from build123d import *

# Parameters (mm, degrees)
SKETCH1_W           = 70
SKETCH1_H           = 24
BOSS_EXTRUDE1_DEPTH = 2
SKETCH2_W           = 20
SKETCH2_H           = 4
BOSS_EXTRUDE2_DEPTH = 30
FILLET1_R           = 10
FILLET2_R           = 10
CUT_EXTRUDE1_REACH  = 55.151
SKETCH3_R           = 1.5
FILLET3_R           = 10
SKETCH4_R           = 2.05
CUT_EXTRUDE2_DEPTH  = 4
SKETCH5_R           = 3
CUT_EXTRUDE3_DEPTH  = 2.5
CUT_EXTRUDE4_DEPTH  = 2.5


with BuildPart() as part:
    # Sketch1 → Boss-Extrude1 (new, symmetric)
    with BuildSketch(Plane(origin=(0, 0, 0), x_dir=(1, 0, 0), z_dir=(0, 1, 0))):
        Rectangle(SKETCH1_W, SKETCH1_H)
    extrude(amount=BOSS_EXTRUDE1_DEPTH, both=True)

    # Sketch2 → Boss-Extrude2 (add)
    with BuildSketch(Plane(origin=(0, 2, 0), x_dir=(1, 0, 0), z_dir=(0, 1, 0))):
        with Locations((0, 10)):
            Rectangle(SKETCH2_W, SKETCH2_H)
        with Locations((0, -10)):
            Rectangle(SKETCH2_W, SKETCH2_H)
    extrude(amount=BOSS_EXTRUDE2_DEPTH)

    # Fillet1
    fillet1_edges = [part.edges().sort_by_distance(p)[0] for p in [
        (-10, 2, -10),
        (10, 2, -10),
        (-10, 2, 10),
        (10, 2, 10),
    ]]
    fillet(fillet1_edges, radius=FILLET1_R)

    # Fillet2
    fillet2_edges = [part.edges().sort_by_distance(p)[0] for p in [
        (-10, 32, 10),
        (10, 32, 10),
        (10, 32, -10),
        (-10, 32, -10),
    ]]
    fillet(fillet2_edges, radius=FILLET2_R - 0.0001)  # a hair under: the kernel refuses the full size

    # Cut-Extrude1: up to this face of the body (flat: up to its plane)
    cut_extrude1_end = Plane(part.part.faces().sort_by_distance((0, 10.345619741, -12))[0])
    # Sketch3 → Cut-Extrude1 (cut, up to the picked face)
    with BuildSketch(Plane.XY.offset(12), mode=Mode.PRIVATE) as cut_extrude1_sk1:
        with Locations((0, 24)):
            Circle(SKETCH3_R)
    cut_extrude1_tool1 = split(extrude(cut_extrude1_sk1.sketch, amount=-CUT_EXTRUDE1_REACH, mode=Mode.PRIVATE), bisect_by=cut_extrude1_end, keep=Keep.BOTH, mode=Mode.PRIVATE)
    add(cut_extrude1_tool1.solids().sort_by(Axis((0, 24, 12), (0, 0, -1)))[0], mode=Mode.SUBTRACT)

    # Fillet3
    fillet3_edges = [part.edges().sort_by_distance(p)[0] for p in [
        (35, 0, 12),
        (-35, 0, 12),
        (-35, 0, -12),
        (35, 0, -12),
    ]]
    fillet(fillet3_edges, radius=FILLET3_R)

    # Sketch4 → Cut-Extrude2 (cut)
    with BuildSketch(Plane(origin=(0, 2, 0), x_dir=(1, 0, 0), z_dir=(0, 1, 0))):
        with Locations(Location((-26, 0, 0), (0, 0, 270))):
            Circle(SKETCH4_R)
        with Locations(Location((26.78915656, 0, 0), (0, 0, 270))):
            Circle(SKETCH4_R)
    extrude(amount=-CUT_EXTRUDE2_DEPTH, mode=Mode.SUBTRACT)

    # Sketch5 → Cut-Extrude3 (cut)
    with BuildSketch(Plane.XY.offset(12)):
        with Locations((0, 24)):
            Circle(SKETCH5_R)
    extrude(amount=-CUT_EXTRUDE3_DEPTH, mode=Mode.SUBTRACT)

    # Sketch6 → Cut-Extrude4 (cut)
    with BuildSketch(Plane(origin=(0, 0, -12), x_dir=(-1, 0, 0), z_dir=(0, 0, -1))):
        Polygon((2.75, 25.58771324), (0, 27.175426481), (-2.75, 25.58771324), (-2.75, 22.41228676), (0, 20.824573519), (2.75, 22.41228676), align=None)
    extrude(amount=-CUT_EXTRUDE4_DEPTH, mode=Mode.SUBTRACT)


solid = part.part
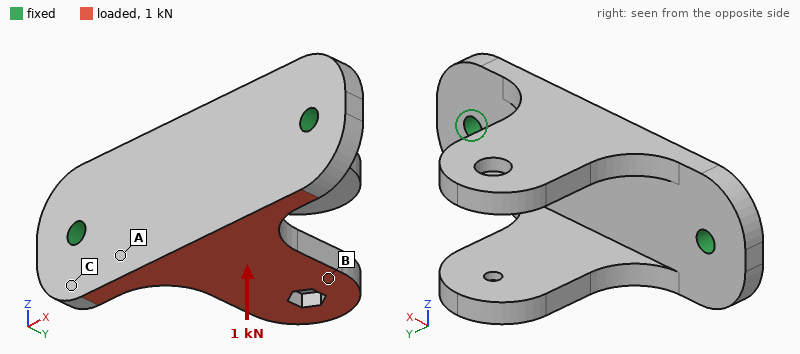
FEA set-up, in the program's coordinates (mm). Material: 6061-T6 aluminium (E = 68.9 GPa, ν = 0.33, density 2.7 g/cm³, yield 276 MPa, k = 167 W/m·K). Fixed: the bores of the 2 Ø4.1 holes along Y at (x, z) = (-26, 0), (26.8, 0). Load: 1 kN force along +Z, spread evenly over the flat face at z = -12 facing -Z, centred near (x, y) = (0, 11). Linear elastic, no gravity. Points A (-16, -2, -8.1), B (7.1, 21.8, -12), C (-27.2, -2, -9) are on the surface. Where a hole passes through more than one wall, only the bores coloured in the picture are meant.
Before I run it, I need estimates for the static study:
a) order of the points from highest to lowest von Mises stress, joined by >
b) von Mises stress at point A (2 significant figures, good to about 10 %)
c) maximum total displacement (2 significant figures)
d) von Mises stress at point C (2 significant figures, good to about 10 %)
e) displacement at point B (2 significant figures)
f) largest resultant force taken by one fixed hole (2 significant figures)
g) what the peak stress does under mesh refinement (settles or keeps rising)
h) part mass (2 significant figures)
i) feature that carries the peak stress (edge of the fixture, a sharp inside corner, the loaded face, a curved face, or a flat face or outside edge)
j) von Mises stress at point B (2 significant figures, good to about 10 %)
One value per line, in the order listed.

A > C > B
78 MPa
0.59 mm
50 MPa
0.38 mm
510 N
keeps rising
29 g
edge of the fixture
20 MPa
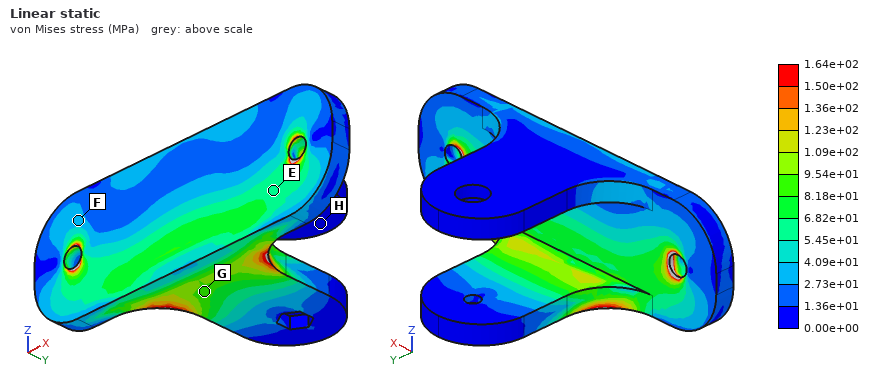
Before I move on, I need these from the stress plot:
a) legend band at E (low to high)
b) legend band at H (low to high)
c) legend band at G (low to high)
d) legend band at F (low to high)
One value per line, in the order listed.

5.45e+01 to 6.82e+01 MPa
0.00e+00 to 1.36e+01 MPa
8.18e+01 to 9.54e+01 MPa
2.73e+01 to 4.09e+01 MPa
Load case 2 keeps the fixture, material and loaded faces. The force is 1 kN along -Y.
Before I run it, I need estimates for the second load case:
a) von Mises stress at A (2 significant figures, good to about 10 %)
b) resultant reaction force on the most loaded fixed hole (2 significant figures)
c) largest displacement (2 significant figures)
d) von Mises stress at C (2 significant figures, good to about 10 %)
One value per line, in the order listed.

56 MPa
570 N
0.29 mm
63 MPa
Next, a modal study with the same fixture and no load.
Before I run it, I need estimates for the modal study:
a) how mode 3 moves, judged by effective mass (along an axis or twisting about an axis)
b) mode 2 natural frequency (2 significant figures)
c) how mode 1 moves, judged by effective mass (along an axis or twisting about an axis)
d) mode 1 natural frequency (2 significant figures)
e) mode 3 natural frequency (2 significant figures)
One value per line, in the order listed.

along Y
3200 Hz
along Z
2500 Hz
6400 Hz
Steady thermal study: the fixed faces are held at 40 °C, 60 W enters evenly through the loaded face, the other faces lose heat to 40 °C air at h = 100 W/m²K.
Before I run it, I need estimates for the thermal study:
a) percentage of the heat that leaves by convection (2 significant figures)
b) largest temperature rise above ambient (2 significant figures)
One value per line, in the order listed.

22 %
74 K
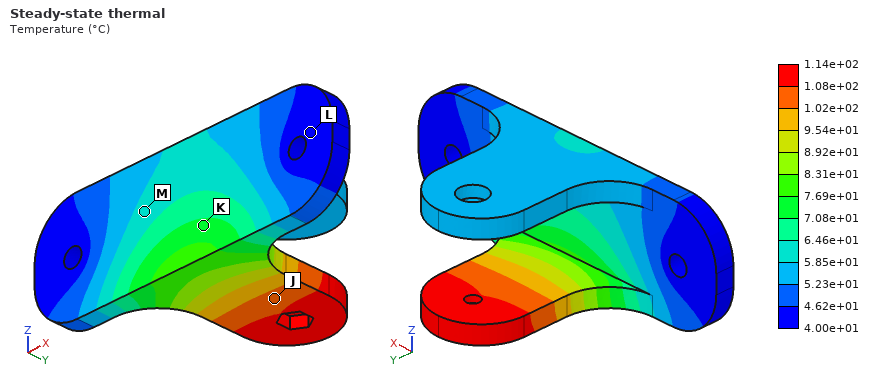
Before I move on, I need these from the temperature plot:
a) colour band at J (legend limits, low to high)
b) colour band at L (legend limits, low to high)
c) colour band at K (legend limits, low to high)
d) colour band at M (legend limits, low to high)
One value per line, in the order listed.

1.02e+02 to 1.08e+02 °C
4.00e+01 to 4.62e+01 °C
7.08e+01 to 7.69e+01 °C
5.85e+01 to 6.46e+01 °C
